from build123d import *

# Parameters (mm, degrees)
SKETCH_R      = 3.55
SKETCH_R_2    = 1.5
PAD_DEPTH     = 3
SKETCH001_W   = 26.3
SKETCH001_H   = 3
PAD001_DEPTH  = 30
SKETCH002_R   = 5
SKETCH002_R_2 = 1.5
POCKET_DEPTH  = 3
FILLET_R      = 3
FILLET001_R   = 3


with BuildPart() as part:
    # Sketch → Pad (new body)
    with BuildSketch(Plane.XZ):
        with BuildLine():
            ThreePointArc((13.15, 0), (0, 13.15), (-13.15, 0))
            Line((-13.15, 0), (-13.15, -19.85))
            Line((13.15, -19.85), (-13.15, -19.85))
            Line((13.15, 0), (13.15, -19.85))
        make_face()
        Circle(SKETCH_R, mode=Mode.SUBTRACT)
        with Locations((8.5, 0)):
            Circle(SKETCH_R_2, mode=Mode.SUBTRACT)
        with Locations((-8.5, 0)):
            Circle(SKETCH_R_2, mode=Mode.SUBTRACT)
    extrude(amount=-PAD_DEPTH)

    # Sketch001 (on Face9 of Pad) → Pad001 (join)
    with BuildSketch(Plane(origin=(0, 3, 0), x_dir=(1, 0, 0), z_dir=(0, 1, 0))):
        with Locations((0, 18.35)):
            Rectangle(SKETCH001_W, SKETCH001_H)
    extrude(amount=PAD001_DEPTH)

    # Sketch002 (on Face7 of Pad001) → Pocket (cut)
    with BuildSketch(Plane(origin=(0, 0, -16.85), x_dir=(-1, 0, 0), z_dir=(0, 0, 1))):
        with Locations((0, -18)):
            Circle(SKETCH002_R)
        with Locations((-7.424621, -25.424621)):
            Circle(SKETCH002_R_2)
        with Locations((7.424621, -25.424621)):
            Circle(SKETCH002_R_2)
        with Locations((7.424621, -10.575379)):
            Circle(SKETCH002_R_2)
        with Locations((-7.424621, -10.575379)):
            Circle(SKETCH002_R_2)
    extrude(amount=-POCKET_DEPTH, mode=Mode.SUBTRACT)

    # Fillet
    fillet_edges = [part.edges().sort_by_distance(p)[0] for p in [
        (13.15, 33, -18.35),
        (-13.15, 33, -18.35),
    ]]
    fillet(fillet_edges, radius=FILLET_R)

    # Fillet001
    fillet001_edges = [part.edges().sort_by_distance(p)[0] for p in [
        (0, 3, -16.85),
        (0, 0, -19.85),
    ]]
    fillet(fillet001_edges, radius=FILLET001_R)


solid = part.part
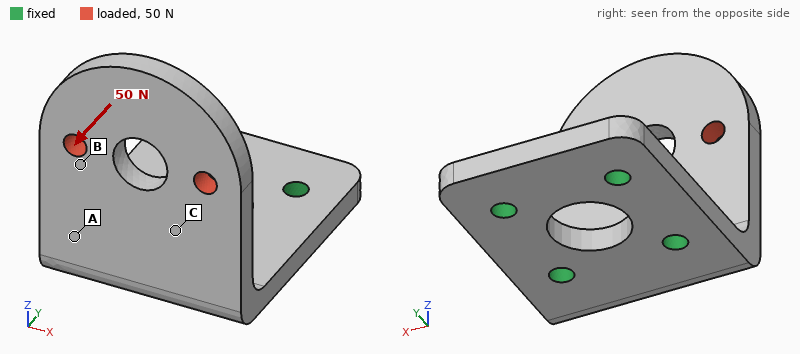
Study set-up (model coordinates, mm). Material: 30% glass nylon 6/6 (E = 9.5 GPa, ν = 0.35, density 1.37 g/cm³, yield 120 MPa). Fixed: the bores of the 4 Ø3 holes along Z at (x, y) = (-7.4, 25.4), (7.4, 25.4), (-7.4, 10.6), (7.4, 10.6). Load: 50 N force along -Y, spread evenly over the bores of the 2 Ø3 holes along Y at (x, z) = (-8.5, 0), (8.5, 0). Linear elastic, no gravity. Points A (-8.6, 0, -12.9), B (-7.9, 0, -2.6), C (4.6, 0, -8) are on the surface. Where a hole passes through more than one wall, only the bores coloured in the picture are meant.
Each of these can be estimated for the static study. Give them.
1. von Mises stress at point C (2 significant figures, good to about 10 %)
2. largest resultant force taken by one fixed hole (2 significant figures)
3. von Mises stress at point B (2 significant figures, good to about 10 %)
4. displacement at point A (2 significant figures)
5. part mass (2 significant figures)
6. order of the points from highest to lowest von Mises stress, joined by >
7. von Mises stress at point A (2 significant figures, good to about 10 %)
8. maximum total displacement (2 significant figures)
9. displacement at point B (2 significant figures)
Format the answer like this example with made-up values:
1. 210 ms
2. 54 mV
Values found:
1. 8.7 MPa
2. 27 N
3. 3.8 MPa
4. 0.11 mm
5. 5.8 g
6. A > C > B
7. 14 MPa
8. 0.62 mm
9. 0.28 mm
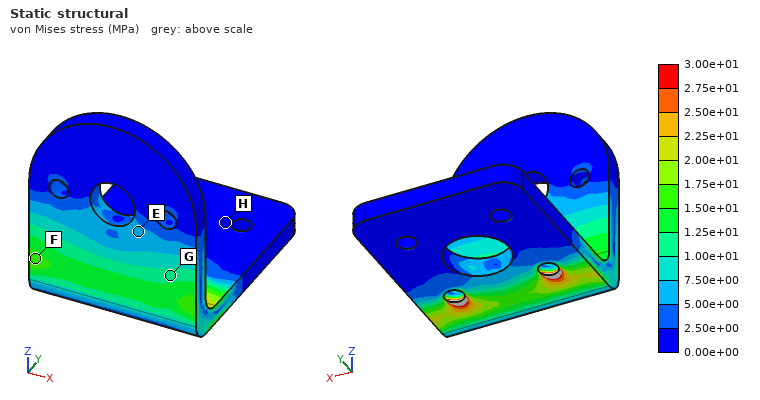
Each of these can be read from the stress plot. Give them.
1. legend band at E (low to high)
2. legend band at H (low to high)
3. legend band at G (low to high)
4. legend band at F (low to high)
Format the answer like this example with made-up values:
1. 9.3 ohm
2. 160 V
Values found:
1. 5.00e+00 to 7.50e+00 MPa
2. 0.00e+00 to 2.50e+00 MPa
3. 1.00e+01 to 1.25e+01 MPa
4. 1.50e+01 to 1.75e+01 MPa
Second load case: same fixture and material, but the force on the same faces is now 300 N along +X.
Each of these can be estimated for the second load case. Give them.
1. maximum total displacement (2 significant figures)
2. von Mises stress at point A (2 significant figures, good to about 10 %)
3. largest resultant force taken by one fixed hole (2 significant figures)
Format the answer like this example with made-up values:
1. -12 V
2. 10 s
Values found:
1. 0.52 mm
2. 16 MPa
3. 380 N
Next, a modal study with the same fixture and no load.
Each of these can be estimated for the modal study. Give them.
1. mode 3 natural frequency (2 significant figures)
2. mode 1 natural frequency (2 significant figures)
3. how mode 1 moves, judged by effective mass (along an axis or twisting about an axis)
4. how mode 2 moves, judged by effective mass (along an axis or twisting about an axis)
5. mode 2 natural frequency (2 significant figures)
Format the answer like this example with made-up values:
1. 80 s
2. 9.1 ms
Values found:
1. 4500 Hz
2. 1200 Hz
3. along Y
4. along X
5. 2800 Hz
